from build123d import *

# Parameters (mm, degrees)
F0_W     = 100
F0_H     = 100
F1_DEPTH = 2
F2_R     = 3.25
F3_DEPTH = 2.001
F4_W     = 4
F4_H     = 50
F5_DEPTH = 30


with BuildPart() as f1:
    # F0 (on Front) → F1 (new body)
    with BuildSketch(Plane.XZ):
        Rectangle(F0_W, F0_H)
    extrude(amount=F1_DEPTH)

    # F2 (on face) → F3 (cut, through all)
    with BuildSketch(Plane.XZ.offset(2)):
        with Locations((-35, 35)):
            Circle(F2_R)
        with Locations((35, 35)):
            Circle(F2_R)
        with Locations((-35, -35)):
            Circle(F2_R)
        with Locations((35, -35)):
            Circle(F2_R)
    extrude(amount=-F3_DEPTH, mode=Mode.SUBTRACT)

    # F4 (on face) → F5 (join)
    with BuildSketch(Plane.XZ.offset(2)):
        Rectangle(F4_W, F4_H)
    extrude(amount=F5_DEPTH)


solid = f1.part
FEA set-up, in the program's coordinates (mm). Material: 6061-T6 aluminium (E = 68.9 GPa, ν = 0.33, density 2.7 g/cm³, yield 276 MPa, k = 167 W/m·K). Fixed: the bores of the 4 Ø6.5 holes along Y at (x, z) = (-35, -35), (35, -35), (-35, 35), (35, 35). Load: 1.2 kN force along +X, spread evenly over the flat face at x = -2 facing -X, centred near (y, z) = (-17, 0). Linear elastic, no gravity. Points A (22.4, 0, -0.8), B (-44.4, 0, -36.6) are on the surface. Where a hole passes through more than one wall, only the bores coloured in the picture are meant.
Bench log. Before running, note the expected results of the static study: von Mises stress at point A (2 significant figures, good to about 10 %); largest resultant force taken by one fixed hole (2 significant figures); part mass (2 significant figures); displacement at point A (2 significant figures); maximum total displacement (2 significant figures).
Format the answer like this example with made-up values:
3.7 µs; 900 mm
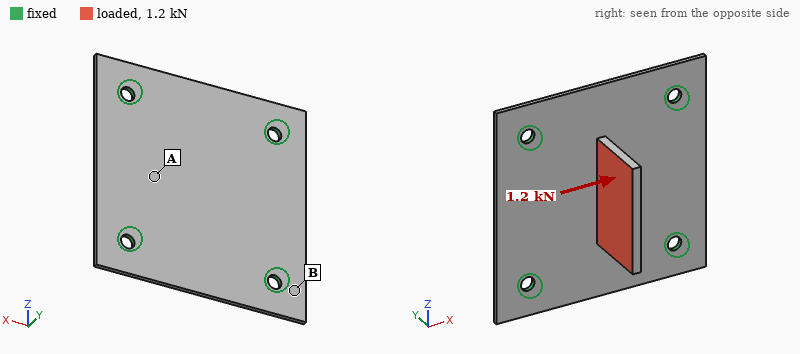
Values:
51 MPa; 370 N; 69 g; 0.22 mm; 1.1 mm
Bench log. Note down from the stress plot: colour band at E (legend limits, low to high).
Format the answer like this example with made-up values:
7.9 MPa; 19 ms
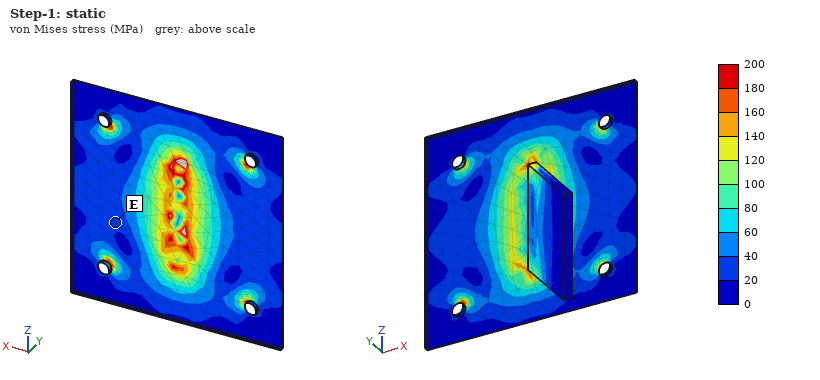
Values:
20 to 40 MPa
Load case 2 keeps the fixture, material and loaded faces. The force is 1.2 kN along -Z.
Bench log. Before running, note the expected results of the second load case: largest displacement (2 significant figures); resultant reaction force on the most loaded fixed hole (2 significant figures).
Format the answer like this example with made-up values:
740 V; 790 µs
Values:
0.41 mm; 360 N
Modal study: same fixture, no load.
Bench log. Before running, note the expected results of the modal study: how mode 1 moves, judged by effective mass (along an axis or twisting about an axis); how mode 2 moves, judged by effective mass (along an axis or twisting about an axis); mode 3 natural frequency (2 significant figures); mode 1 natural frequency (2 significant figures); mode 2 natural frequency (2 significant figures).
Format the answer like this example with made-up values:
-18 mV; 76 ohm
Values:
along Y; along X; 1800 Hz; 1300 Hz; 1600 Hz
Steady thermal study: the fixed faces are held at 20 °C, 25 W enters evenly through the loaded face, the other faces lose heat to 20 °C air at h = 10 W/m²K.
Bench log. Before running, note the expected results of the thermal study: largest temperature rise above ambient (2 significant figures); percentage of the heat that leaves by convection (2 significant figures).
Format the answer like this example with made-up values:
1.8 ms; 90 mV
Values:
31 K; 8.5 %
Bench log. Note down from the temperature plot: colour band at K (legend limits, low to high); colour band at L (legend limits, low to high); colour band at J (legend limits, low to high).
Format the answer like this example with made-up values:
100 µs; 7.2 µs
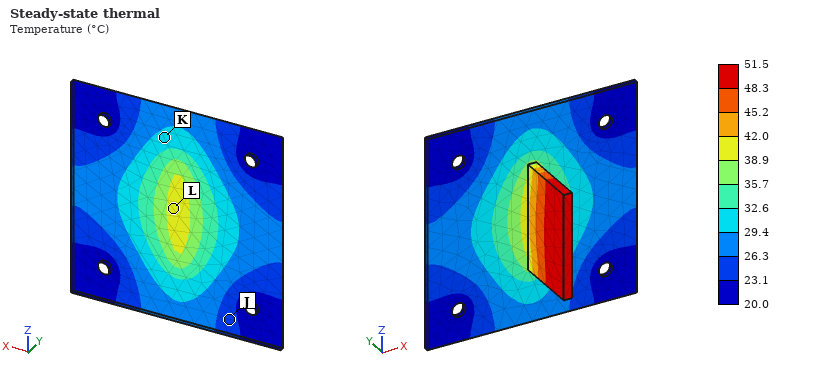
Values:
29.4 to 32.6 °C; 38.9 to 42.0 °C; 23.1 to 26.3 °C
